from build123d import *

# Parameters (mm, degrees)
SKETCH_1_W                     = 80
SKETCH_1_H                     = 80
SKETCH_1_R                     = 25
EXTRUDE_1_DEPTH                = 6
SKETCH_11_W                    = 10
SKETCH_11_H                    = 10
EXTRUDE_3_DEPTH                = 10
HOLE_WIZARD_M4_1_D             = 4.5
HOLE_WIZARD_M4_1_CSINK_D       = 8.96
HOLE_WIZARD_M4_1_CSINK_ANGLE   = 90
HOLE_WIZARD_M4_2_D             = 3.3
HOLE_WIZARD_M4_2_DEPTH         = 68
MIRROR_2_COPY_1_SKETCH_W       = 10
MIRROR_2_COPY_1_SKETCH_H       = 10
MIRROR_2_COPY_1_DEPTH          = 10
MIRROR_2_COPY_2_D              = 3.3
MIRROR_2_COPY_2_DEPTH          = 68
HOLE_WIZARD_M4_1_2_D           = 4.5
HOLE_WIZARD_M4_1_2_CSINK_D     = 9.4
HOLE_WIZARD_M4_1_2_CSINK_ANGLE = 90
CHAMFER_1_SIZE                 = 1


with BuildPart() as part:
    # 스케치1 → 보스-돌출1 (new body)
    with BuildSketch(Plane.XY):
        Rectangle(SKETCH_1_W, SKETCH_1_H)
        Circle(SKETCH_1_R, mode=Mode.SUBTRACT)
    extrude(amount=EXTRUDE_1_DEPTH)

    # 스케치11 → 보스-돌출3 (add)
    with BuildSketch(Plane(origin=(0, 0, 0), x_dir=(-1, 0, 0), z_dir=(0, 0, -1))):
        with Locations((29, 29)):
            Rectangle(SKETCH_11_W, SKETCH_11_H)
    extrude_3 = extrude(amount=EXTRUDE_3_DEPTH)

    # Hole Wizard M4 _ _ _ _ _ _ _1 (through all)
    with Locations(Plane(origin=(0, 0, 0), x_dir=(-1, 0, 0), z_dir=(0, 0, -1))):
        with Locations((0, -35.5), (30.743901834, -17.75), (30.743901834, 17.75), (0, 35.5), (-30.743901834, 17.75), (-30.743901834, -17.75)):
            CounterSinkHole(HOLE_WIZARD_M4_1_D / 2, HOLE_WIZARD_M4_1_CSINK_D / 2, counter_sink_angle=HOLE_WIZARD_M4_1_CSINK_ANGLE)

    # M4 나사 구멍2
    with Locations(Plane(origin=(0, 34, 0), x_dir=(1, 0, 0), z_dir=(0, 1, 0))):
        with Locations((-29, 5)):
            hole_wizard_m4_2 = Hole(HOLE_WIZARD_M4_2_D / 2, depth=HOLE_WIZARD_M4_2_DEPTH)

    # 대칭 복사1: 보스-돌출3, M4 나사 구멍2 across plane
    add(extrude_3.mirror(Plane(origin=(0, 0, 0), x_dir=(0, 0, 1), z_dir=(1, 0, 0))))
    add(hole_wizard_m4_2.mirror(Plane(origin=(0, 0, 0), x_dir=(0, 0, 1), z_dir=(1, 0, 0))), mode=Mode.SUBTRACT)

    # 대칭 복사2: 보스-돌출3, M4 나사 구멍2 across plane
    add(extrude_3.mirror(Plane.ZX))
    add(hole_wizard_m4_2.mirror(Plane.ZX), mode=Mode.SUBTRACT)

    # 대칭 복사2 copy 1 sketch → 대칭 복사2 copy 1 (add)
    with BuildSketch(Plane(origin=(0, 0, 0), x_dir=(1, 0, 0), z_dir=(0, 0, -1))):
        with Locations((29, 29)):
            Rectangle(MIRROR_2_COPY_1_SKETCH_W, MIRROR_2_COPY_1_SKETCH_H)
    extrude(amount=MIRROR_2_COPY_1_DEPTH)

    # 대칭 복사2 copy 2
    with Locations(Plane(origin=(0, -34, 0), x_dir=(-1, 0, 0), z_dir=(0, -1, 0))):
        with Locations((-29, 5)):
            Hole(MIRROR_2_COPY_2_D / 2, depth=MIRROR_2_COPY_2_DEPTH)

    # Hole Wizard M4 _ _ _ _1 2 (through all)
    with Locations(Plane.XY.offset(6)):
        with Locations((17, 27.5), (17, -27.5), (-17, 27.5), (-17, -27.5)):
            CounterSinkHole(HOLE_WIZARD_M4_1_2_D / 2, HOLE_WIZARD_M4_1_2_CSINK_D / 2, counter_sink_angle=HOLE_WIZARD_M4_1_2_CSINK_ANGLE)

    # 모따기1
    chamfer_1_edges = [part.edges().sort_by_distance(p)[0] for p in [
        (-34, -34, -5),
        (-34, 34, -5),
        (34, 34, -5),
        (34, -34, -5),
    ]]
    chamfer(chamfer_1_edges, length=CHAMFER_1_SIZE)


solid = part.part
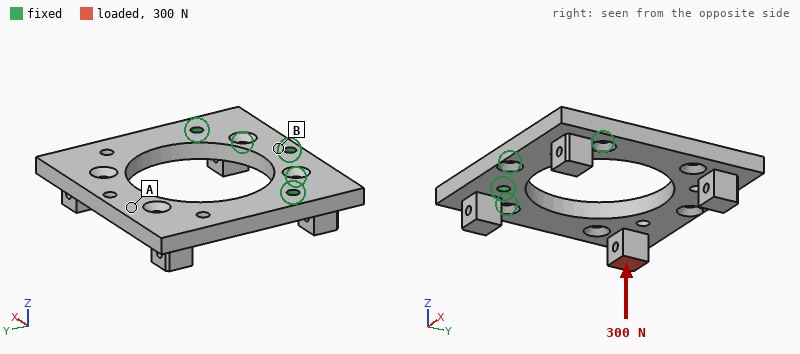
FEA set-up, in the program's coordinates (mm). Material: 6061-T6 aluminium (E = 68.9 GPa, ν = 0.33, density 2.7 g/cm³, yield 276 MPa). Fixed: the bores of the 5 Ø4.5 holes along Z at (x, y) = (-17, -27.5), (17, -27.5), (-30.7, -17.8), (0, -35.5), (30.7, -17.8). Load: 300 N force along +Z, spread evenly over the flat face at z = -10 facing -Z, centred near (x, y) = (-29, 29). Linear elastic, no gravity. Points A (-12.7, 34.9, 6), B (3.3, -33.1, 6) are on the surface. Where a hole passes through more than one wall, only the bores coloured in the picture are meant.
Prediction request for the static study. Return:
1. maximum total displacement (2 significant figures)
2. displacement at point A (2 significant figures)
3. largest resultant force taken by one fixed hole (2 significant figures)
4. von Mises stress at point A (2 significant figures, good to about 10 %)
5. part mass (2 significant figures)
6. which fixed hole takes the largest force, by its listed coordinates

0.51 mm
0.38 mm
500 N
18 MPa
78 g
(-30.7, -17.8)
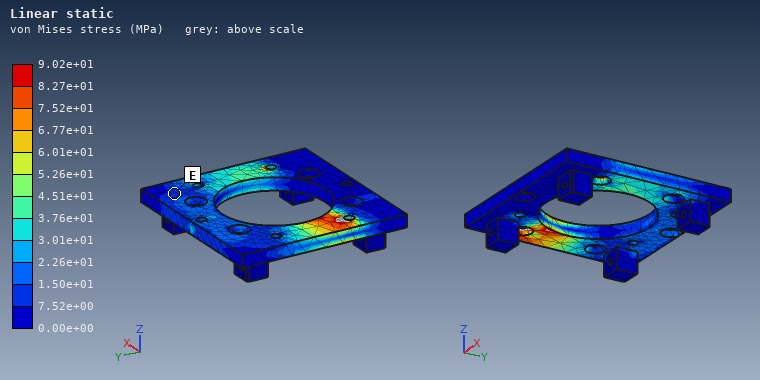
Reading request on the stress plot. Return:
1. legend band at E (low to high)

7.52e+00 to 1.50e+01 MPa
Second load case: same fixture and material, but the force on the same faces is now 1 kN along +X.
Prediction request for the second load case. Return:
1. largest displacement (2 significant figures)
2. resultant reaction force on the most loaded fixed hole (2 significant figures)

0.25 mm
1.1 kN
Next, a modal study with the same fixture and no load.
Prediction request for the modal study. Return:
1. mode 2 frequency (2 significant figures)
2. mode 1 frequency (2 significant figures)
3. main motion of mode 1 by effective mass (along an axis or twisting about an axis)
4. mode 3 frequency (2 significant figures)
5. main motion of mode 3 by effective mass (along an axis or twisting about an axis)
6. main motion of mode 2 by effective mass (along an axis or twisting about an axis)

1900 Hz
880 Hz
along Z
4400 Hz
along X
twisting about Y
